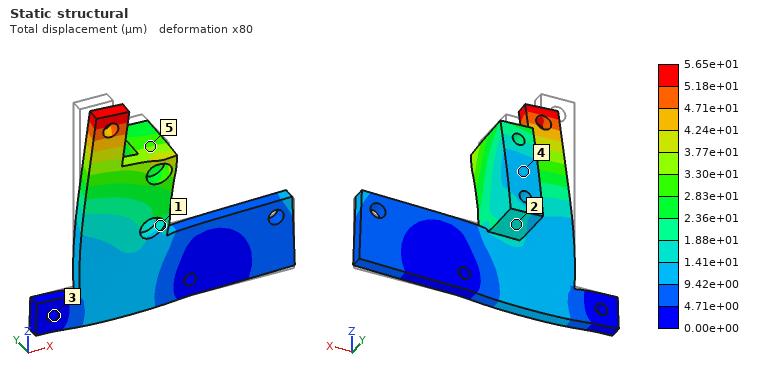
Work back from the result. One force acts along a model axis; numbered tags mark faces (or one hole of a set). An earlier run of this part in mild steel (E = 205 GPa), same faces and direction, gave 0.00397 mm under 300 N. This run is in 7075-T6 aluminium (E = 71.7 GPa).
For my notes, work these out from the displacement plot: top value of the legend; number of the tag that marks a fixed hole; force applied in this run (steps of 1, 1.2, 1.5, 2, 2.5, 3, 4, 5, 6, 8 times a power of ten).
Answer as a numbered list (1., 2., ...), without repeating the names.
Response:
1. 5.65e+01 µm
2. 3
3. 1.5 kN
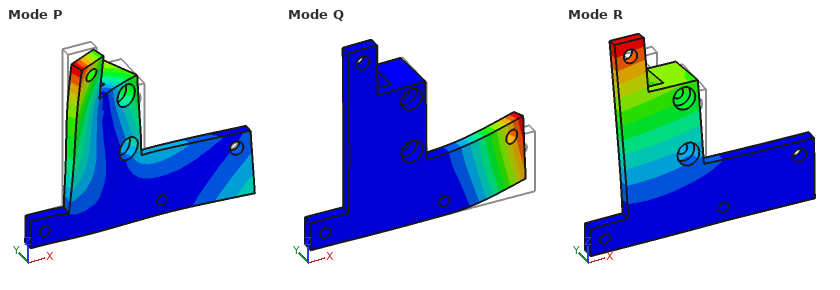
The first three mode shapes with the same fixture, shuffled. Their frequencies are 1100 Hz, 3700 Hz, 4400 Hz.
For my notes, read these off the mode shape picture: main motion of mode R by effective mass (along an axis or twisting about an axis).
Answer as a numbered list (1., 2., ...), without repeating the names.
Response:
1. along Y
